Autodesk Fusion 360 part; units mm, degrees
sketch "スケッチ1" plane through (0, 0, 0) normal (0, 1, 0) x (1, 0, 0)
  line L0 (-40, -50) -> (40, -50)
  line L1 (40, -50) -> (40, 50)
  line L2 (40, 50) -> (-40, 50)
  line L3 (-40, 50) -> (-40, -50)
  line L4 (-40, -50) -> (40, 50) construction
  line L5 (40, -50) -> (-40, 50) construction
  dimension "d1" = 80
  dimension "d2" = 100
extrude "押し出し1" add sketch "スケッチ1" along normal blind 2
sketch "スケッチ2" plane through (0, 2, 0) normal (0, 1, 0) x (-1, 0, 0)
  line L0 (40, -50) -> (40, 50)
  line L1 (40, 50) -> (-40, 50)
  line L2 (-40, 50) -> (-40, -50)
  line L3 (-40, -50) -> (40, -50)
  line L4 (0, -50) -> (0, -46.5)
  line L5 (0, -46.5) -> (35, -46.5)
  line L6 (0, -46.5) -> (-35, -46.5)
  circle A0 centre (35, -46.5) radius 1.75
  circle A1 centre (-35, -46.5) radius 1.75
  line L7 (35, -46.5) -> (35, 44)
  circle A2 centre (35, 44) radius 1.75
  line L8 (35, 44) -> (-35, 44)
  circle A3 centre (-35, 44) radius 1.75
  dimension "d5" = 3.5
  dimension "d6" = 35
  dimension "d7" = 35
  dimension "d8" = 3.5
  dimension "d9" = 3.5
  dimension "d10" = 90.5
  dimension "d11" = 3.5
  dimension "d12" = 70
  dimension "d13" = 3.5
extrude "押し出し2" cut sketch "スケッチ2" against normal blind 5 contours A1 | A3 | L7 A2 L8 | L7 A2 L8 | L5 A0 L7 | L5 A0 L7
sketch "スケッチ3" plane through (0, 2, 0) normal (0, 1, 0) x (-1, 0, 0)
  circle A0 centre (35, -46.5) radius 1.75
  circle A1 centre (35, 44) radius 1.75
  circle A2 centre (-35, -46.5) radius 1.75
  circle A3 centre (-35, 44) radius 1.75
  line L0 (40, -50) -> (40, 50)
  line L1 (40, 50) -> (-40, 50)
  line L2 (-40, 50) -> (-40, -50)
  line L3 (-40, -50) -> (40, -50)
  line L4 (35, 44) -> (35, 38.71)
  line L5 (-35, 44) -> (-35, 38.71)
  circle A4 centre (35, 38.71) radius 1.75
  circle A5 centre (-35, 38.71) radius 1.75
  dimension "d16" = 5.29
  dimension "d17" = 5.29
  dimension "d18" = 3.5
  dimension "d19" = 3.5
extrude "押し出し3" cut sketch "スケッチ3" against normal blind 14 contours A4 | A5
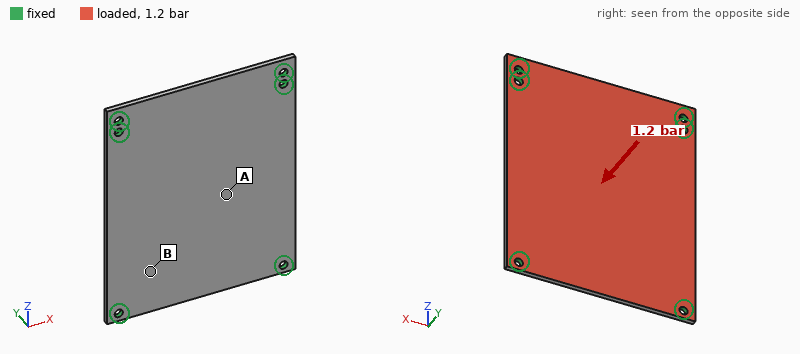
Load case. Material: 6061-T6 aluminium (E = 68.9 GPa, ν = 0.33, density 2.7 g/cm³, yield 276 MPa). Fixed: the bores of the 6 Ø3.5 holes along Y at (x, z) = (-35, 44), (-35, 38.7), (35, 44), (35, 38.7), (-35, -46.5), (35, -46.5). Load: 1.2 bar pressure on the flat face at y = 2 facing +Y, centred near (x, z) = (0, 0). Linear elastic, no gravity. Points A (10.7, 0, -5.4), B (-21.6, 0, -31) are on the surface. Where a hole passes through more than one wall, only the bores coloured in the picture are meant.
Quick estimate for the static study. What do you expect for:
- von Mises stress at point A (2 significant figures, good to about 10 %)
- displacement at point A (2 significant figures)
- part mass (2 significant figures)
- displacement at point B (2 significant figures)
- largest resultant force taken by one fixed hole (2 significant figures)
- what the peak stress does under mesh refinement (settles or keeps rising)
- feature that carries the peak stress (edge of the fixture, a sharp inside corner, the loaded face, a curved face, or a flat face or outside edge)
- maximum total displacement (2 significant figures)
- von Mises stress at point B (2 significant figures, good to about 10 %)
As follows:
62 MPa
0.67 mm
43 g
0.34 mm
340 N
keeps rising
edge of the fixture
0.70 mm
23 MPa
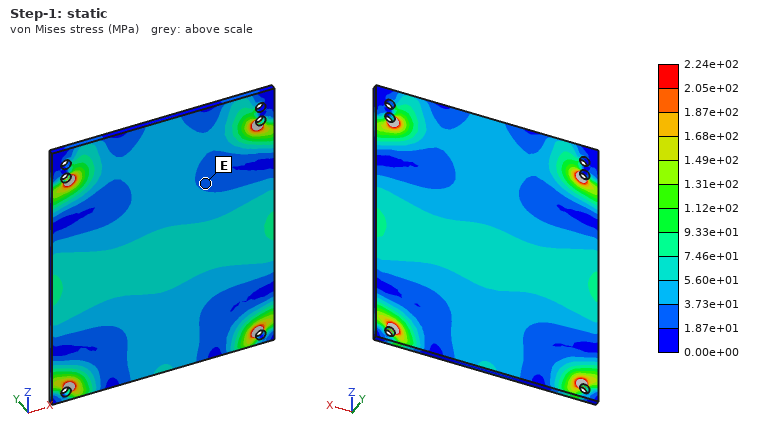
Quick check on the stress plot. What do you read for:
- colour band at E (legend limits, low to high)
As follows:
1.87e+01 to 3.73e+01 MPa
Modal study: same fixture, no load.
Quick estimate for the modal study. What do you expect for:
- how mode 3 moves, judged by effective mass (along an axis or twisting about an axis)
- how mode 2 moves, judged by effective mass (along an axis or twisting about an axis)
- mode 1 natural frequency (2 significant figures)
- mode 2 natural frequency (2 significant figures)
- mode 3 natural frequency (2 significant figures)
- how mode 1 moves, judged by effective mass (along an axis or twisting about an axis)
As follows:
twisting about X
twisting about Z
1100 Hz
1700 Hz
2200 Hz
along Y
